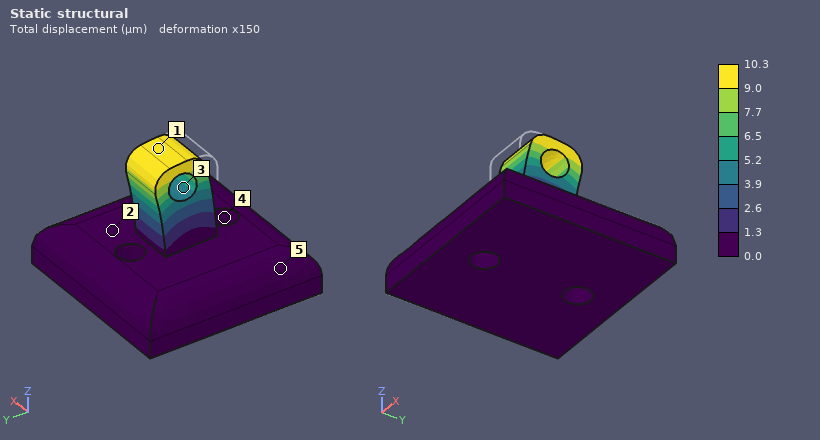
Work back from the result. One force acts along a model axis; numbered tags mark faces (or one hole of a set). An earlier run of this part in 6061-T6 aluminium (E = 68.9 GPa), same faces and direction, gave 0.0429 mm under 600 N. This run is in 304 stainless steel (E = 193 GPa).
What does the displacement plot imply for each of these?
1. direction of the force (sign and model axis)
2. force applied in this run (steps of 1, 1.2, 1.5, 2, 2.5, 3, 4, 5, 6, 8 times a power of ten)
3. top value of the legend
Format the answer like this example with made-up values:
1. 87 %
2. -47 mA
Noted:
1. +Y
2. 400 N
3. 10.3 µm
